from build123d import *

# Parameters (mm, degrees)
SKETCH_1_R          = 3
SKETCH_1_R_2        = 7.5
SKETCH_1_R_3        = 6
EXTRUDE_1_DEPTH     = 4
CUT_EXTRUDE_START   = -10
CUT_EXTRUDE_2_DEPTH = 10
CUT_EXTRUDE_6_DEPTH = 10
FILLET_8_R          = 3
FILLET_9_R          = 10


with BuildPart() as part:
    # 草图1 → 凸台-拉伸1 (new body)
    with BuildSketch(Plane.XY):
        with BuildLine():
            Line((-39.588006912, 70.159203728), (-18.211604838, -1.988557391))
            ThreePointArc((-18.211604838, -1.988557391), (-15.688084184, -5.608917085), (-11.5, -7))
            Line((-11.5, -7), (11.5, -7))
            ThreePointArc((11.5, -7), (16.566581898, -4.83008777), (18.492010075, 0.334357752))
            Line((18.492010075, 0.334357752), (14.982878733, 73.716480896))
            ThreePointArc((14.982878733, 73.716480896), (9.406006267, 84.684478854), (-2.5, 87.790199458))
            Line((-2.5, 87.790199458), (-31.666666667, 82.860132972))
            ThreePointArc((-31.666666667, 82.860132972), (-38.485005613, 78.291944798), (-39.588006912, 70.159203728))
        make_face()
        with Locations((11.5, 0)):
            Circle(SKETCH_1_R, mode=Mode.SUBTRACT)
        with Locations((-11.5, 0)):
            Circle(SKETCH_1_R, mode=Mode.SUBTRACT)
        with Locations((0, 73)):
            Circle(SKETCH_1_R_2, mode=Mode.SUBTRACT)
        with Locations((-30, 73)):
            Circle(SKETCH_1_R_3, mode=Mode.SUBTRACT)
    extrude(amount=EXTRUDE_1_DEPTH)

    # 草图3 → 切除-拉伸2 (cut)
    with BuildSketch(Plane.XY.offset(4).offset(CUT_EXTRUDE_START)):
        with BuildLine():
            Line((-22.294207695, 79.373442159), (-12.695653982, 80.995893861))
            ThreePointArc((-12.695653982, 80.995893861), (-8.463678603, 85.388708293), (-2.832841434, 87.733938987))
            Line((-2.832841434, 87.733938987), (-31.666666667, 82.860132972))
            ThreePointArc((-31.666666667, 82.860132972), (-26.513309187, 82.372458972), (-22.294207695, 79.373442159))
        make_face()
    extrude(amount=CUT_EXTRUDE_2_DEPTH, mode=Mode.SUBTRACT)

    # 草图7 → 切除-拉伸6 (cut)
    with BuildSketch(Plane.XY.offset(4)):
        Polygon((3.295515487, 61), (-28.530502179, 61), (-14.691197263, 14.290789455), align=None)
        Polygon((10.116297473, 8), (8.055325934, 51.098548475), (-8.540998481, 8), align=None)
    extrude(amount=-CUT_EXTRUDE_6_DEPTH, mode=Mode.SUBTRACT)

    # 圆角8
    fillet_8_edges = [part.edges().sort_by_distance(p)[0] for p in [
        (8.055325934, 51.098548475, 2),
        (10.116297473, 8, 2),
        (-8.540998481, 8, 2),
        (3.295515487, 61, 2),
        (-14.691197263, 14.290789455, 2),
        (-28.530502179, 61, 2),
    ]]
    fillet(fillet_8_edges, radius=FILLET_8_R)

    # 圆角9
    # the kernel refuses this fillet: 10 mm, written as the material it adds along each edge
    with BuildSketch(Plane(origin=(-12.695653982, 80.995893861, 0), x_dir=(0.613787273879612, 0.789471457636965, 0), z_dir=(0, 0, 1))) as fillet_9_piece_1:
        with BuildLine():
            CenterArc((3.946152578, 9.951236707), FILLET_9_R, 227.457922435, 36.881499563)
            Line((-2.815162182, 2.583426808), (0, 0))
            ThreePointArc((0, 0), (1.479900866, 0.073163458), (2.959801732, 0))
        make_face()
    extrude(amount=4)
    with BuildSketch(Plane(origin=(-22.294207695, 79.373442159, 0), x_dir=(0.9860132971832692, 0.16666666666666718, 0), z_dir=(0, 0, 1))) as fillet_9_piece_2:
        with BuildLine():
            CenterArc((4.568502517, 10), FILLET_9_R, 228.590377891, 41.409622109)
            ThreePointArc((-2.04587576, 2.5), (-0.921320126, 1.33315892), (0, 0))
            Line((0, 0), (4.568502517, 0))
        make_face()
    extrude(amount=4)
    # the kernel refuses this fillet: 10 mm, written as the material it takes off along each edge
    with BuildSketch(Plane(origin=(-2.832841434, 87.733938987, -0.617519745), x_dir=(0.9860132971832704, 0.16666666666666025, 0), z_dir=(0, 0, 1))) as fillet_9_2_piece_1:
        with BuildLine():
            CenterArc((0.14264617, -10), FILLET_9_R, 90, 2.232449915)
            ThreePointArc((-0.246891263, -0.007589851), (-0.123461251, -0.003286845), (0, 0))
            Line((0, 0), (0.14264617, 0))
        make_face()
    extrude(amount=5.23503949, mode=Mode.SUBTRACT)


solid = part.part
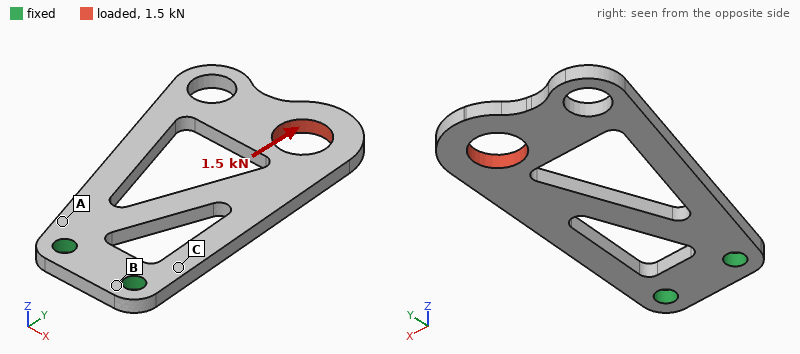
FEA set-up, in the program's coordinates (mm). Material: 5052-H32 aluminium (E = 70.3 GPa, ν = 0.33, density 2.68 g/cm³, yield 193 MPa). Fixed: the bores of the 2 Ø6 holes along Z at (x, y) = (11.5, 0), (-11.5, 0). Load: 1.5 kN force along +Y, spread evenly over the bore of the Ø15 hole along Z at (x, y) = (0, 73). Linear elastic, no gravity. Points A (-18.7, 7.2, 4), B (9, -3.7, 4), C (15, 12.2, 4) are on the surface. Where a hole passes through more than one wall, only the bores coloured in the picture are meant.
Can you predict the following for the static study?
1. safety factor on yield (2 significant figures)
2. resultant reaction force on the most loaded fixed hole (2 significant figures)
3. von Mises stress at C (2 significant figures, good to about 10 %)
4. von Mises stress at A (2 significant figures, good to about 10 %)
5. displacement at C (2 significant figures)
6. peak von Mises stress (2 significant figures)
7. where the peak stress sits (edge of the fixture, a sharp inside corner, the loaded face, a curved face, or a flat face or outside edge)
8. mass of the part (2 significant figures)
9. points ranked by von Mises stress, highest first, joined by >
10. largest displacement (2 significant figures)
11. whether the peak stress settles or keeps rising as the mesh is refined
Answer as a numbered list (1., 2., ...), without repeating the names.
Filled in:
1. 2.4
2. 760 N
3. 22 MPa
4. 12 MPa
5. 5.6 µm
6. 81 MPa
7. a curved face
8. 30 g
9. C > A > B
10. 36 µm
11. settles
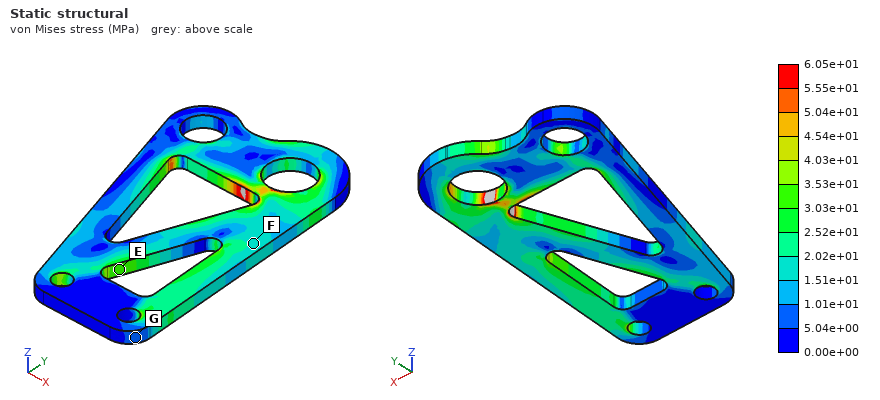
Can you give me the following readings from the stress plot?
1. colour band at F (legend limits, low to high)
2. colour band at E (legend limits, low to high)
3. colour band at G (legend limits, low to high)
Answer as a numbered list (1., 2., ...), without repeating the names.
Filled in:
1. 1.51e+01 to 2.02e+01 MPa
2. 3.03e+01 to 3.53e+01 MPa
3. 5.04e+00 to 1.01e+01 MPa
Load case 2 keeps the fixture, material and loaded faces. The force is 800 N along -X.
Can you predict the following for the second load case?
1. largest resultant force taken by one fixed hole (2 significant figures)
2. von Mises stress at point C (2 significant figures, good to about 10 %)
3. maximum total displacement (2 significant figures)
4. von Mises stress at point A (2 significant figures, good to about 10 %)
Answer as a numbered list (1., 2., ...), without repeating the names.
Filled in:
1. 2.0 kN
2. 61 MPa
3. 0.22 mm
4. 46 MPa
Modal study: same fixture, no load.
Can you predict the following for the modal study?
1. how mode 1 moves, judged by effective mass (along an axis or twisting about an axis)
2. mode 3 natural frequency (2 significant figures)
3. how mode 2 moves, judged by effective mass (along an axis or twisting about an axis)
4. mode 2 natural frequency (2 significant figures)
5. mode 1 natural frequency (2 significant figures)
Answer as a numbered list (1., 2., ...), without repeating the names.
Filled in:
1. along Z
2. 2700 Hz
3. twisting about Y
4. 1200 Hz
5. 400 Hz
